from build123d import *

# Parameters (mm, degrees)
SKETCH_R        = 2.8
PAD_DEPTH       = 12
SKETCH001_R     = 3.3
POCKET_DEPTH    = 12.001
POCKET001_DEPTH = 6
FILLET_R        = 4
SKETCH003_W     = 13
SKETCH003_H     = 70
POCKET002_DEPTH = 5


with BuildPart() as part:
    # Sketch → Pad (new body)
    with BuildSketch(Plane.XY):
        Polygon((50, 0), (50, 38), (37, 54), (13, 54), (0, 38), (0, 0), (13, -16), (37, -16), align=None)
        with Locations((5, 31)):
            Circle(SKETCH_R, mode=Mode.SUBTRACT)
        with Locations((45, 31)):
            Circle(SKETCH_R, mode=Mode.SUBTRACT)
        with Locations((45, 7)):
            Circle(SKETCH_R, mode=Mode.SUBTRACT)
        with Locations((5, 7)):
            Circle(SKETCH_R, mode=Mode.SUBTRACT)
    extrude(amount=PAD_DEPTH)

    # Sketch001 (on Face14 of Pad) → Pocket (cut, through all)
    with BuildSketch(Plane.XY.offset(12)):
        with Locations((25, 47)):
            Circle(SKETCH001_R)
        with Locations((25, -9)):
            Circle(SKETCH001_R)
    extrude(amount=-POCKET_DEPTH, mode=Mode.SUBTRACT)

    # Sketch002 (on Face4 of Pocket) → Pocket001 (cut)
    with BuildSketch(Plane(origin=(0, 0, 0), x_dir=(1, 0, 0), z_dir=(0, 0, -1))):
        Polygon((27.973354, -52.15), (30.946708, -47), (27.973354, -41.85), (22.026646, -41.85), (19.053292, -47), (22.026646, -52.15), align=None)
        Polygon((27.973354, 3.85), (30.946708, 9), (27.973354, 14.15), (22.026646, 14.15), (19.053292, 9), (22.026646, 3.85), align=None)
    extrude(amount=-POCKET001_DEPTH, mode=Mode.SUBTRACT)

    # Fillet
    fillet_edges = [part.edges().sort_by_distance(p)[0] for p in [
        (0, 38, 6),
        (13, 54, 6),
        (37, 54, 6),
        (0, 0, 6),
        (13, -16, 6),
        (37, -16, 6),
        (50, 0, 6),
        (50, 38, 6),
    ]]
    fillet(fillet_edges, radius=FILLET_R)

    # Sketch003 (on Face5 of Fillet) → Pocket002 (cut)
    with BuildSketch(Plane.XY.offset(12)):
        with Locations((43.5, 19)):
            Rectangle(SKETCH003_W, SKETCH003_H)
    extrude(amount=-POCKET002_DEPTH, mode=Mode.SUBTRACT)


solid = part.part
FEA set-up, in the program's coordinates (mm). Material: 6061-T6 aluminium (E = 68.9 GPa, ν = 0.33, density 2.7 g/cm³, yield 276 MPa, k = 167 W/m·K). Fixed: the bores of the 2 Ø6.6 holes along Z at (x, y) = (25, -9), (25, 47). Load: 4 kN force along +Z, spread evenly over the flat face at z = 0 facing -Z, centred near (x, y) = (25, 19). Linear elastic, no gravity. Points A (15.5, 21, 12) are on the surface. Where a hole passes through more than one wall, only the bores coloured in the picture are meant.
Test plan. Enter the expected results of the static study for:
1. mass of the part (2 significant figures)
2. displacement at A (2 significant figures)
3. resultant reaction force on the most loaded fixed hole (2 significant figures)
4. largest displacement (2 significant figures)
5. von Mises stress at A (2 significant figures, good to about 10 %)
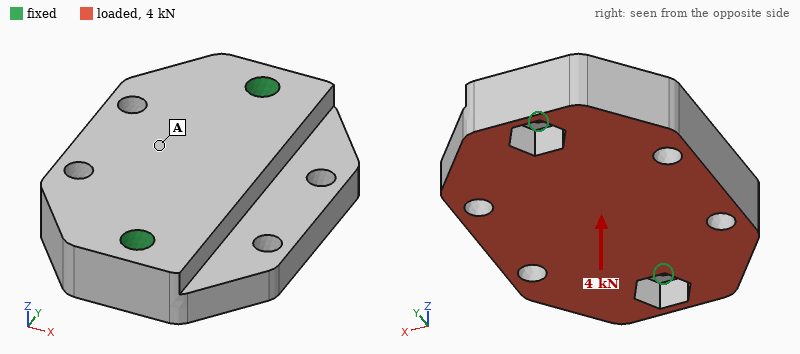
84 g
15 µm
2.3 kN
27 µm
13 MPa
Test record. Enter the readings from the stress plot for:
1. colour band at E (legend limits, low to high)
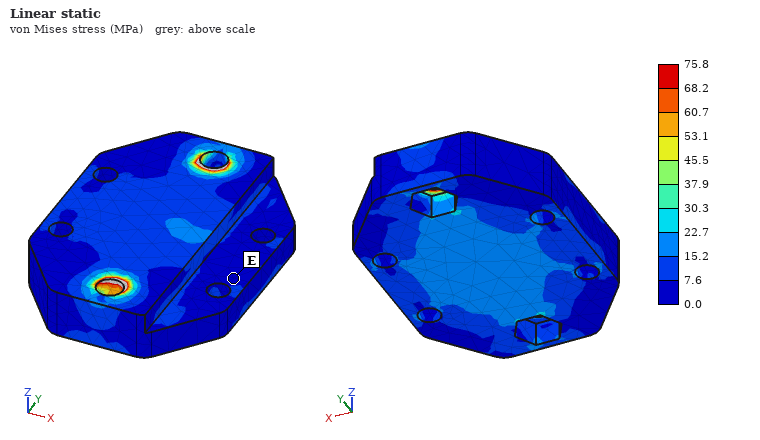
0.0 to 7.6 MPa
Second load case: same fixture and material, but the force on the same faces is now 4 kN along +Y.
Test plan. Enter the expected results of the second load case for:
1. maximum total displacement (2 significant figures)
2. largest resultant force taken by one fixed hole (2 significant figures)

4.4 µm
2.1 kN
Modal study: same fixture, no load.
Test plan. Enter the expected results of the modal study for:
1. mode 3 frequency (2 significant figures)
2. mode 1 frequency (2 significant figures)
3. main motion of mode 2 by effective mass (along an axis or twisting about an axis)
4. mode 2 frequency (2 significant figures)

16 kHz
6100 Hz
along Z
9500 Hz
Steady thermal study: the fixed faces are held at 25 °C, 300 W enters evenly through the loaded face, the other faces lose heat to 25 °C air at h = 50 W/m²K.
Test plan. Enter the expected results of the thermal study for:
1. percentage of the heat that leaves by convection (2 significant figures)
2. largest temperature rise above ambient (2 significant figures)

3.8 %
54 K
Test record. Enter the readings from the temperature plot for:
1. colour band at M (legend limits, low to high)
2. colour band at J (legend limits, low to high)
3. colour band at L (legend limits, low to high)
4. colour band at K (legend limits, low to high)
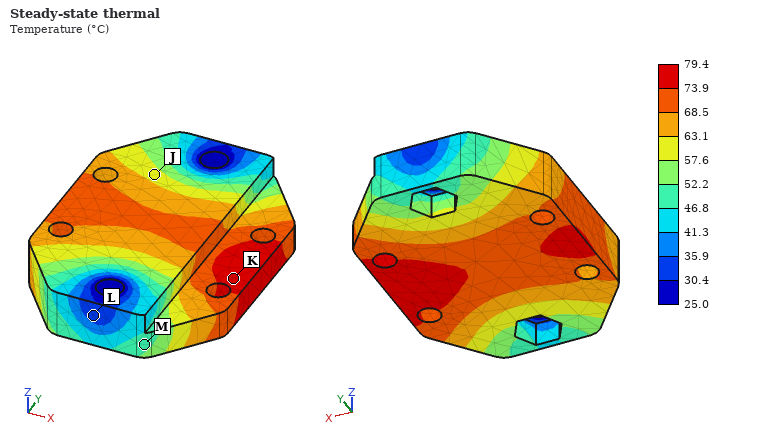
46.8 to 52.2 °C
57.6 to 63.1 °C
30.4 to 35.9 °C
73.9 to 79.4 °C
